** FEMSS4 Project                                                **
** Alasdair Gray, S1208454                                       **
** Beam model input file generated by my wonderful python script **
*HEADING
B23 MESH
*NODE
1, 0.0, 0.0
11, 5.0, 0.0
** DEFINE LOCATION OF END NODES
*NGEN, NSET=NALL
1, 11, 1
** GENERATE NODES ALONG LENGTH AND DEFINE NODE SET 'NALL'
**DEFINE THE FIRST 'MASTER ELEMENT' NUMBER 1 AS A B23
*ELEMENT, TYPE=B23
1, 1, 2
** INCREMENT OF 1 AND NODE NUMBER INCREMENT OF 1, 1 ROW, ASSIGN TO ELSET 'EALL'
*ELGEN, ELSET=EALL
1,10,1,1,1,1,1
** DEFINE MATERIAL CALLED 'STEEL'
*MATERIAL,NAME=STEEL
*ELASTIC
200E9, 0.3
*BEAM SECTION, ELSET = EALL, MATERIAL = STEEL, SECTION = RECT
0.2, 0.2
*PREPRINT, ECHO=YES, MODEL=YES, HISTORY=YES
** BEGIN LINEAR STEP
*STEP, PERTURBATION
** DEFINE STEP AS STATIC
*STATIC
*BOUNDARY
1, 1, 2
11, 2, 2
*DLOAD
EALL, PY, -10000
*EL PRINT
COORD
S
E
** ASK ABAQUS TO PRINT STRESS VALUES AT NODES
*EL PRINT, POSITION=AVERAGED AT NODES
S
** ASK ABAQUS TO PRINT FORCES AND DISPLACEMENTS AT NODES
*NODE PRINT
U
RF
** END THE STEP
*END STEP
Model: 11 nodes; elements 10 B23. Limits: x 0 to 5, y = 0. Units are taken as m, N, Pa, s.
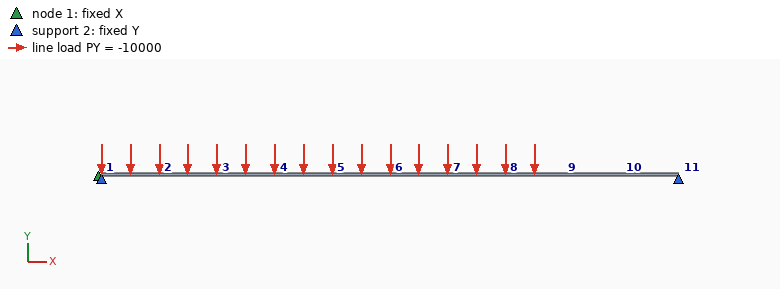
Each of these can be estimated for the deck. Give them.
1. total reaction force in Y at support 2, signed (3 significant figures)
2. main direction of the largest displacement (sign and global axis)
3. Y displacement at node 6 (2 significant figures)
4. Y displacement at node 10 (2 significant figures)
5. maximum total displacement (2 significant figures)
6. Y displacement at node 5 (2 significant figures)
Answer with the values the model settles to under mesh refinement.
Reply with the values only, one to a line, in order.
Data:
50000 N
-Y
-0.0031 m
-9.6e-04 m
0.0031 m
-0.0029 m
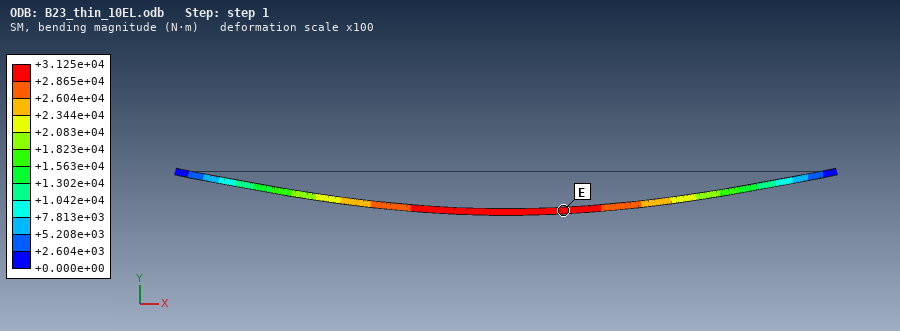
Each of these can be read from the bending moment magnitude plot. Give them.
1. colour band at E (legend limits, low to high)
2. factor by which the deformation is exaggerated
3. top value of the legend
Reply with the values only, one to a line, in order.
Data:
+2.865e+04 to +3.125e+04 N·m
100
+3.125e+04 N·m
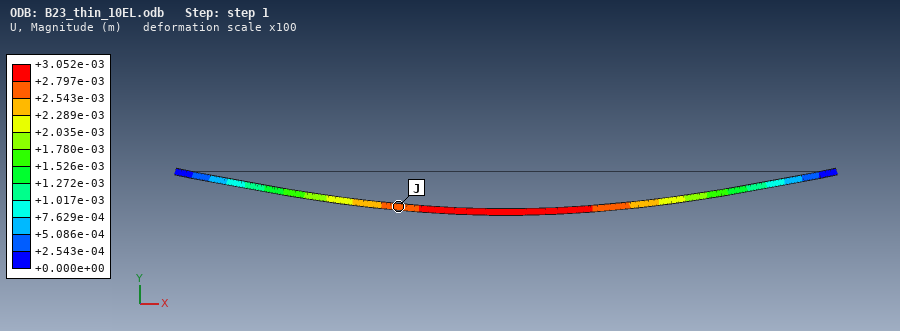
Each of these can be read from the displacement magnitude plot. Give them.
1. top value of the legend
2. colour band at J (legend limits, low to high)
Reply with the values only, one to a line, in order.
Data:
+3.052e-03 m
+2.543e-03 to +2.797e-03 m
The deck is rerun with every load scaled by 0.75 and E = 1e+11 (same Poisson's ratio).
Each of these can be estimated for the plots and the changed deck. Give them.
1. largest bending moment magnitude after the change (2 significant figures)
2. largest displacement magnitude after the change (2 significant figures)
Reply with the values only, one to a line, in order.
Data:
23000 N·m
0.0046 m
